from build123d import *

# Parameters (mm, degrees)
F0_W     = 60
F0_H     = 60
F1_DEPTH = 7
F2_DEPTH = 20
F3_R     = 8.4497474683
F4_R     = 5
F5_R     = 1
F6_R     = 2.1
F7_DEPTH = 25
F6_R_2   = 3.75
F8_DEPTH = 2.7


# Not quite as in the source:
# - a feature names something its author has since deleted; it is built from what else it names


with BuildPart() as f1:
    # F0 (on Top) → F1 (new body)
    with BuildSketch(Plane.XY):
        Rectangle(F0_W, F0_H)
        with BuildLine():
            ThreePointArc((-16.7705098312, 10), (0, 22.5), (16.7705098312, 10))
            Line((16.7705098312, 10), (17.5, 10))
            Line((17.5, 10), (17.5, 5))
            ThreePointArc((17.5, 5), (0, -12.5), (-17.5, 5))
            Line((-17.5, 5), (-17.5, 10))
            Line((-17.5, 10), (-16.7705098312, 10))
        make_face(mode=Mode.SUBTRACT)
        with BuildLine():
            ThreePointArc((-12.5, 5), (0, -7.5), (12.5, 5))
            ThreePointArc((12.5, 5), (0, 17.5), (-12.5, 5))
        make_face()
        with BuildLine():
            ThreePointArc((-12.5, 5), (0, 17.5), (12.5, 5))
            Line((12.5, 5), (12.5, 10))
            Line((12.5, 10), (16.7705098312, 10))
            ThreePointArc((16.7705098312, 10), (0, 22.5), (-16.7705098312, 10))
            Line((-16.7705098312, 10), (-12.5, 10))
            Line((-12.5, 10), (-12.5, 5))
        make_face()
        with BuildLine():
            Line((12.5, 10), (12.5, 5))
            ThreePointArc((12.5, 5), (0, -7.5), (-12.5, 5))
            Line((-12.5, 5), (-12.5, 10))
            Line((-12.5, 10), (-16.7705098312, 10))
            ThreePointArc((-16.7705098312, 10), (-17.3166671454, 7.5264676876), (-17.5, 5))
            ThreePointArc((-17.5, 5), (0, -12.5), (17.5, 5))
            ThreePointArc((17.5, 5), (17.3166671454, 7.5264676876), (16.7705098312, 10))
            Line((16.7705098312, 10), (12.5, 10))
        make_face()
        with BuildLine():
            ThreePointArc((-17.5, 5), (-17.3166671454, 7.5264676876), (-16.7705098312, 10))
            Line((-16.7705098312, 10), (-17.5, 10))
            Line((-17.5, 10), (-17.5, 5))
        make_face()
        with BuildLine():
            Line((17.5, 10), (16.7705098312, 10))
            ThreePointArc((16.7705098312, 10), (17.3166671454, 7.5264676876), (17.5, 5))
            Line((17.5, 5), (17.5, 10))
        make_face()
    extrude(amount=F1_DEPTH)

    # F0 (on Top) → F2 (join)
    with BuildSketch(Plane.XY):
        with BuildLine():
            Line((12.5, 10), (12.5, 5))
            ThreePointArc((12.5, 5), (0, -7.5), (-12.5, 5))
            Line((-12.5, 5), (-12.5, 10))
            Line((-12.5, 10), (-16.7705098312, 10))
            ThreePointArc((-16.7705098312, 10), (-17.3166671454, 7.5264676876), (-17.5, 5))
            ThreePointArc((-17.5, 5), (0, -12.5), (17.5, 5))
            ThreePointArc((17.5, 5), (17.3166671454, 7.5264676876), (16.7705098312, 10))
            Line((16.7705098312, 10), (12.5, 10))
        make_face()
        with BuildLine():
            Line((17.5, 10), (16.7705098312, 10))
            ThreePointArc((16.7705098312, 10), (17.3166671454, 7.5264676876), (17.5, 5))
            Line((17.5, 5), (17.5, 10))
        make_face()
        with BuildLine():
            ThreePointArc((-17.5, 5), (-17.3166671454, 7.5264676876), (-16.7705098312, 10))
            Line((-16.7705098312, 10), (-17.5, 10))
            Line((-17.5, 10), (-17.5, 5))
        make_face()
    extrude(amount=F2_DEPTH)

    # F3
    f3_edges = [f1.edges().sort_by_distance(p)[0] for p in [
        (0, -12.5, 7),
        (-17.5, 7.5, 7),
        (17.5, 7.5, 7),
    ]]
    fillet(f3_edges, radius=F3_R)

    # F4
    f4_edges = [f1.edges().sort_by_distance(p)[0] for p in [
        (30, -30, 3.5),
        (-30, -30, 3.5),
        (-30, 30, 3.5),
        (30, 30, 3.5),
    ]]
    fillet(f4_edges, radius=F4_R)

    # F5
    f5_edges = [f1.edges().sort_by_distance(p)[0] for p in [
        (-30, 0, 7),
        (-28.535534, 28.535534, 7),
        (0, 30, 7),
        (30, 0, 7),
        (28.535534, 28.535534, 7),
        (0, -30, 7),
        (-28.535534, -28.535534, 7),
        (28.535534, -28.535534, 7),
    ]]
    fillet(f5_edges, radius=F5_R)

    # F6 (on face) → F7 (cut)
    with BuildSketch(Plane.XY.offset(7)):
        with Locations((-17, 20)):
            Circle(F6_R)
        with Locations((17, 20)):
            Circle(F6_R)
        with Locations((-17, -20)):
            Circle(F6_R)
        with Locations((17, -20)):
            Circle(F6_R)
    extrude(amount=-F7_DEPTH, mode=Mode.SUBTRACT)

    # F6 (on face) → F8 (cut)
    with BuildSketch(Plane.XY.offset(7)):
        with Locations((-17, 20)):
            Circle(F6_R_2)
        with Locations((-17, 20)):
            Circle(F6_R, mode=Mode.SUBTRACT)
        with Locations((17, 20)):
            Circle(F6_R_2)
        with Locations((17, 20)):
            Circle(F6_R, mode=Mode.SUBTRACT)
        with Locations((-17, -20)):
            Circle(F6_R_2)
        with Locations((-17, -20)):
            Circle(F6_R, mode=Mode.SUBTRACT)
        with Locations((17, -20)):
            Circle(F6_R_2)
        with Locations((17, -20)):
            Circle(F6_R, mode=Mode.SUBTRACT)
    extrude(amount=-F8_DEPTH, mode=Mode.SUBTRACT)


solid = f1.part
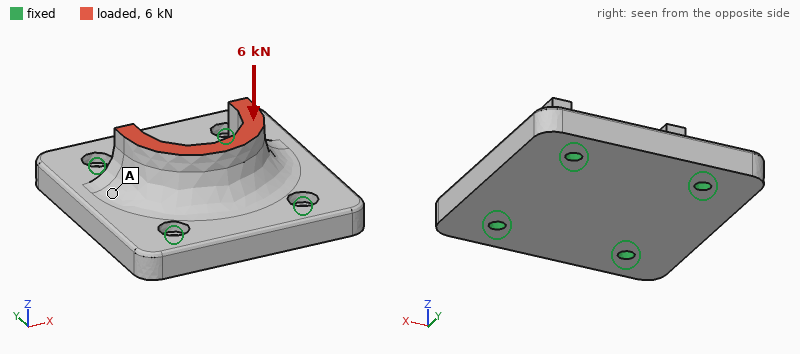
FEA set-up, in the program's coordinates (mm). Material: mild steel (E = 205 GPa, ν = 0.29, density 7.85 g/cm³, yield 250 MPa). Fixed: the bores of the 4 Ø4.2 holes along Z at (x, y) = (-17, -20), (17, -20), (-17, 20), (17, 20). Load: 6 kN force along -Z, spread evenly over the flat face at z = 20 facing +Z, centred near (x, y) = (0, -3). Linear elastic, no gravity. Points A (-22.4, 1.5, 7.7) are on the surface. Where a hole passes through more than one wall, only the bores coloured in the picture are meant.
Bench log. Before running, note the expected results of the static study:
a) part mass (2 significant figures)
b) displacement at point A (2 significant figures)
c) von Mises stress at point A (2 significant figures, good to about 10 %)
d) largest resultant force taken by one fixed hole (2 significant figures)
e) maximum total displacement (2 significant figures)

230 g
5.9 µm
21 MPa
2.0 kN
7.7 µm
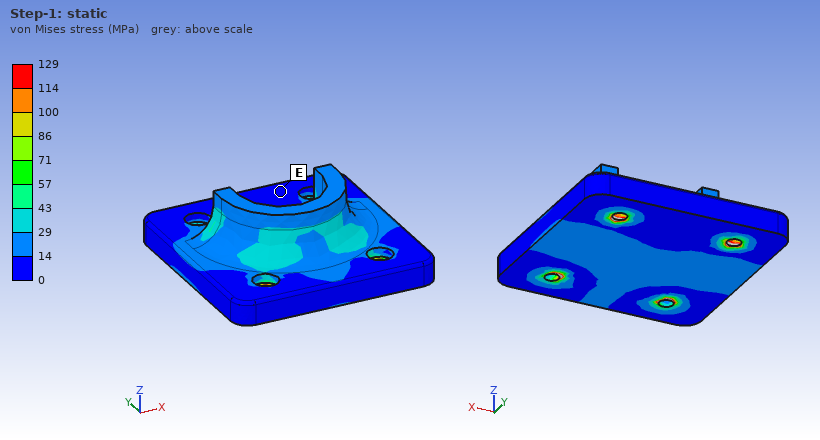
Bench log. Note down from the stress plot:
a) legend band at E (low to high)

0 to 14 MPa
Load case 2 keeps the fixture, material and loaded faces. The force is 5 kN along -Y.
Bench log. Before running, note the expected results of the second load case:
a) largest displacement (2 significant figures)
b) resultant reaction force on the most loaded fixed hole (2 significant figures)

14 µm
1.8 kN
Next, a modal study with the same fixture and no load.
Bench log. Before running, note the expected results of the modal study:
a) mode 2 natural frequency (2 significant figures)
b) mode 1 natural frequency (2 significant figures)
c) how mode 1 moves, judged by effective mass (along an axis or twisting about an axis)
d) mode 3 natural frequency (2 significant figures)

14 kHz
13 kHz
along Z
17 kHz
